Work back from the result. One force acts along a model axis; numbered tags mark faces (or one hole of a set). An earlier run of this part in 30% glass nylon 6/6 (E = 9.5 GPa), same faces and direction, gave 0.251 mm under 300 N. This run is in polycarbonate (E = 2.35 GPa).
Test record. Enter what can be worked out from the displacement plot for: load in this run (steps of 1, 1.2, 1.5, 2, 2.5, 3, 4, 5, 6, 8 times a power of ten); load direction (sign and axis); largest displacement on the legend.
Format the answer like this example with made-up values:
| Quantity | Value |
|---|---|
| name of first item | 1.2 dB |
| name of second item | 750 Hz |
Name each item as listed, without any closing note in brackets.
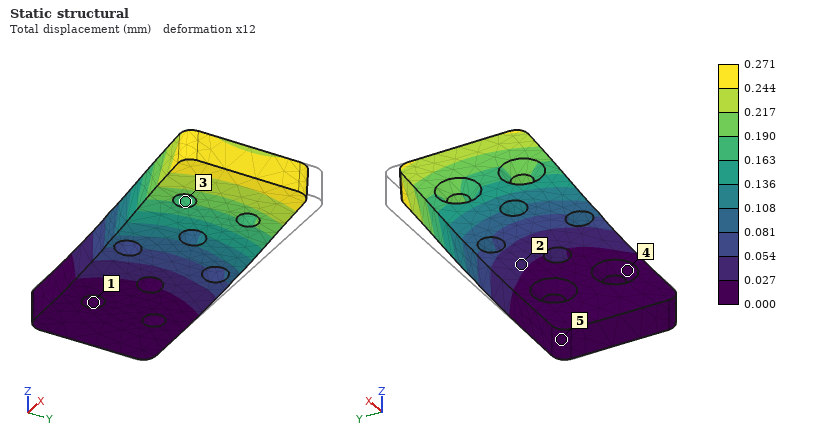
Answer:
| Quantity | Value |
|---|---|
| load in this run | 80 N |
| load direction | -Y |
| largest displacement on the legend | 0.271 mm |
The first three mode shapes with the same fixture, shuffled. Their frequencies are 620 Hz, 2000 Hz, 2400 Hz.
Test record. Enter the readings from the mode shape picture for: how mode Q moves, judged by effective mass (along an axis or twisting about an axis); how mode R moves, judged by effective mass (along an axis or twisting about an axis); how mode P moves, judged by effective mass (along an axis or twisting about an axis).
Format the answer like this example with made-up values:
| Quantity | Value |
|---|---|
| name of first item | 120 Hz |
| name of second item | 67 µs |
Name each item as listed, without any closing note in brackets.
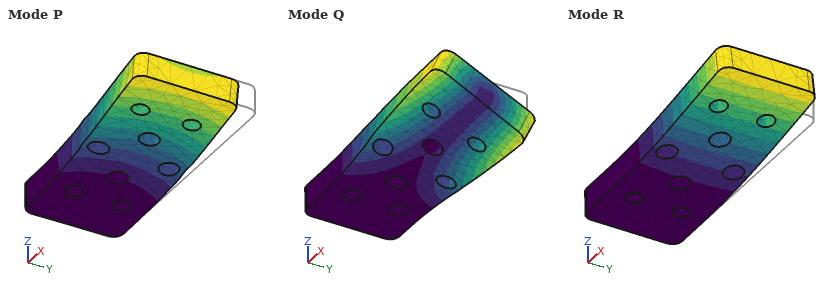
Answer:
| Quantity | Value |
|---|---|
| how mode Q moves, judged by effective mass | twisting about X |
| how mode R moves, judged by effective mass | along Z |
| how mode P moves, judged by effective mass | along Y |
